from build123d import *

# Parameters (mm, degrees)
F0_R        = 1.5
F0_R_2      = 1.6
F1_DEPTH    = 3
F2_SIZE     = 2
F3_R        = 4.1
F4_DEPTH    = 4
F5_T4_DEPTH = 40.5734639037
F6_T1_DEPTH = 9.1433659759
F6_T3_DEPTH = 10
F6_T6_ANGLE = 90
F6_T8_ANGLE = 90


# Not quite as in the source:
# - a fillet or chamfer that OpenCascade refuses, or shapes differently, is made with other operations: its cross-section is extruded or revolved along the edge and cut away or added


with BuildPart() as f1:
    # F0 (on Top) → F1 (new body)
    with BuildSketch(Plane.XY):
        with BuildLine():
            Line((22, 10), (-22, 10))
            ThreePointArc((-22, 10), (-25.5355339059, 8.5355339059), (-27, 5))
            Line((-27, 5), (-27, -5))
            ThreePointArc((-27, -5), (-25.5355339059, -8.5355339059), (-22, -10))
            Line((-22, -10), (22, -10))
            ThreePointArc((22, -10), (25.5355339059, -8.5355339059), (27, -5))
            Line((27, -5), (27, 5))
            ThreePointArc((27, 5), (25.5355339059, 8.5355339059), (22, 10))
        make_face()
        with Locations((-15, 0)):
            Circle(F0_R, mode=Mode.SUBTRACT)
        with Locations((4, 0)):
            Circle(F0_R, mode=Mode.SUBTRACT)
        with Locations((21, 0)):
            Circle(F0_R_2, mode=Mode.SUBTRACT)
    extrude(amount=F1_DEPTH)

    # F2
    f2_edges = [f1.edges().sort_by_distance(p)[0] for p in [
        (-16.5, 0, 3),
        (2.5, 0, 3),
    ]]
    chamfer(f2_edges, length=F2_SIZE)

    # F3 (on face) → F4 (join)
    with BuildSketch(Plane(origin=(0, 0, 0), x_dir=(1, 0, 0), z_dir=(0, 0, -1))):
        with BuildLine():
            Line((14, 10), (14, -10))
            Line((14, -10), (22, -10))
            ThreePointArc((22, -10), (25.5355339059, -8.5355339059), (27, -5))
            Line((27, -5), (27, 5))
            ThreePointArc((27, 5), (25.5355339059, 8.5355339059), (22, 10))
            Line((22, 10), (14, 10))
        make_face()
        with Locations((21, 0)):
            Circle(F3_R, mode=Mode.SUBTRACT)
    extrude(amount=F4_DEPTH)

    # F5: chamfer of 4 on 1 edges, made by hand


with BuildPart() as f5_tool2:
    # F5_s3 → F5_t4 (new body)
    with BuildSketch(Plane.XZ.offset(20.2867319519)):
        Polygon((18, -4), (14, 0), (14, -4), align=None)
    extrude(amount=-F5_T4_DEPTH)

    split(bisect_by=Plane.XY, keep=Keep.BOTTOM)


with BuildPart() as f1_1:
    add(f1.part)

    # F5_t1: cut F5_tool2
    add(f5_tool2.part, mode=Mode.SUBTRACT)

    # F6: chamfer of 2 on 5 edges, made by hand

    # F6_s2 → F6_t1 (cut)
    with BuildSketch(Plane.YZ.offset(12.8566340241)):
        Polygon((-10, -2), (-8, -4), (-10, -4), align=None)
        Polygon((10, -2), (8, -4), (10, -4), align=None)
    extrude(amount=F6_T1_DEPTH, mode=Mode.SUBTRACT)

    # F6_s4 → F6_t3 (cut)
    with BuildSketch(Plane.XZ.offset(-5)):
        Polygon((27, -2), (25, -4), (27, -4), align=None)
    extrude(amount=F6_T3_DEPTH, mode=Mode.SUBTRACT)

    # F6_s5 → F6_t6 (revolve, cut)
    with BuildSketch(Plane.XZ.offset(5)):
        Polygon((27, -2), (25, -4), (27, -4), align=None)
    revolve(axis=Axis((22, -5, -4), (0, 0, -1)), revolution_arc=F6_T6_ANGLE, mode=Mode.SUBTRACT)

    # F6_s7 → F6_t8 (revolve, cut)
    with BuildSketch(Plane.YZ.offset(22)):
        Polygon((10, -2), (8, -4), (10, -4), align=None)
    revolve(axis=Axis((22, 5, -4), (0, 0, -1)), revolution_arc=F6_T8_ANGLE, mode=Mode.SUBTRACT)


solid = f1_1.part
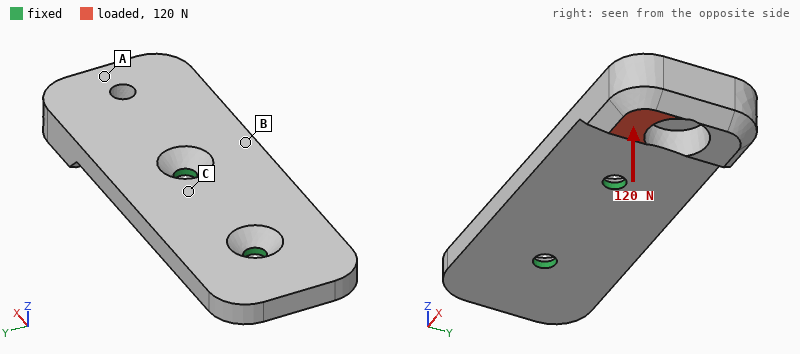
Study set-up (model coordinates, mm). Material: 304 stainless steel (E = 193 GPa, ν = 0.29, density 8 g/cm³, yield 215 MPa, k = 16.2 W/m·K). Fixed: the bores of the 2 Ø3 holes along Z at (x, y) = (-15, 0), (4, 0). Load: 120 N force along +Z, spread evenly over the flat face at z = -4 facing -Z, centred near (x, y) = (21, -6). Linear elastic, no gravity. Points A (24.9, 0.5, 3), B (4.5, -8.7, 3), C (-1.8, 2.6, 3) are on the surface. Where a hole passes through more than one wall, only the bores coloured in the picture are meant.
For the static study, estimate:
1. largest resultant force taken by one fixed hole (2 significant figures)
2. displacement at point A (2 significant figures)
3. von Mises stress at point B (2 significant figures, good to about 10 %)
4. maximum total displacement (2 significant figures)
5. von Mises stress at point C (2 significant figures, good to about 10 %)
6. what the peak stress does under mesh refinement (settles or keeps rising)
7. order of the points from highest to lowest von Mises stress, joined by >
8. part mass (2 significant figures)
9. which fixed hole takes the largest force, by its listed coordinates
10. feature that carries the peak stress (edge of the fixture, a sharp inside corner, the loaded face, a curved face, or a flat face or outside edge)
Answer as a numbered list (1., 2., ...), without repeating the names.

1. 320 N
2. 48 µm
3. 63 MPa
4. 61 µm
5. 24 MPa
6. keeps rising
7. B > C > A
8. 29 g
9. (4, 0)
10. edge of the fixture
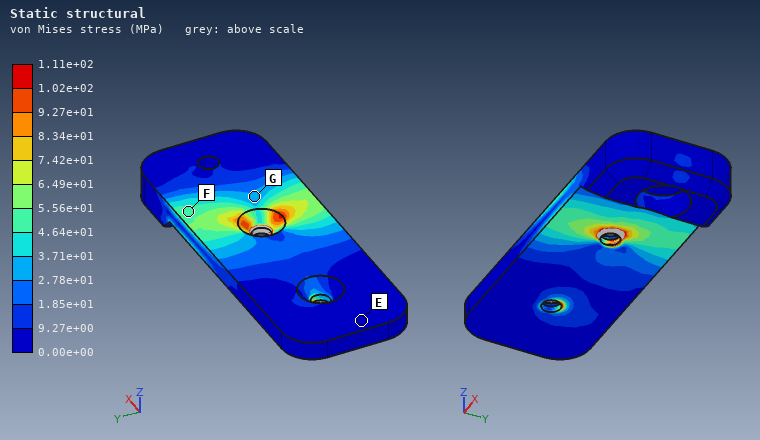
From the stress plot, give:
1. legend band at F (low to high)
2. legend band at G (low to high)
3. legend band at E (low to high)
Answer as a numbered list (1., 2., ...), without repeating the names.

1. 4.64e+01 to 5.56e+01 MPa
2. 2.78e+01 to 3.71e+01 MPa
3. 0.00e+00 to 9.27e+00 MPa
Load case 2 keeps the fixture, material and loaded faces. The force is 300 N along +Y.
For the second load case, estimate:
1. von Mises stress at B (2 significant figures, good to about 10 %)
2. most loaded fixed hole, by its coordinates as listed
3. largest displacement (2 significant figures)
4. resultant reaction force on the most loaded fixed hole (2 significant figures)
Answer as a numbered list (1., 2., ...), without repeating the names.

1. 43 MPa
2. (4, 0)
3. 25 µm
4. 550 N
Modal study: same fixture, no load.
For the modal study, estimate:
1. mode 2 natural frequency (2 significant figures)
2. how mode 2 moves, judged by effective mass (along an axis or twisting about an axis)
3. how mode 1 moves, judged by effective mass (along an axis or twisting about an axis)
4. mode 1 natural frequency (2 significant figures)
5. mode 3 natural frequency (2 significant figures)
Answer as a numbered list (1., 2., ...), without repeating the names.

1. 5500 Hz
2. twisting about X
3. along Z
4. 2800 Hz
5. 10 kHz
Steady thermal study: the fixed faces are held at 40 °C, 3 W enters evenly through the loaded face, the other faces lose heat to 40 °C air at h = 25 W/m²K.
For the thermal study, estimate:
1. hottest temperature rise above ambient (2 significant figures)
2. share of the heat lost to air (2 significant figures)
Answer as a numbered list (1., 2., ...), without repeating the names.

1. 66 K
2. 39 %
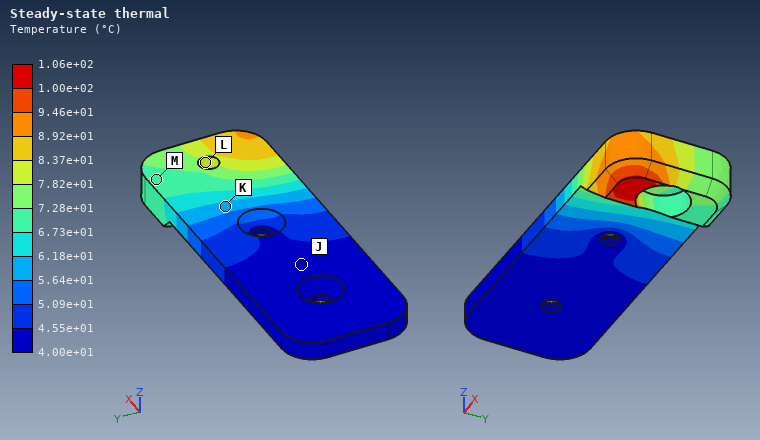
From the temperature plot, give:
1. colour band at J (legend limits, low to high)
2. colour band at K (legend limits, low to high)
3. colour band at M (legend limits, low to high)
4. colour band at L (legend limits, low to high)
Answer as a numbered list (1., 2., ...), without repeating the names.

1. 4.00e+01 to 4.55e+01 °C
2. 5.64e+01 to 6.18e+01 °C
3. 6.73e+01 to 7.28e+01 °C
4. 7.82e+01 to 8.37e+01 °C
